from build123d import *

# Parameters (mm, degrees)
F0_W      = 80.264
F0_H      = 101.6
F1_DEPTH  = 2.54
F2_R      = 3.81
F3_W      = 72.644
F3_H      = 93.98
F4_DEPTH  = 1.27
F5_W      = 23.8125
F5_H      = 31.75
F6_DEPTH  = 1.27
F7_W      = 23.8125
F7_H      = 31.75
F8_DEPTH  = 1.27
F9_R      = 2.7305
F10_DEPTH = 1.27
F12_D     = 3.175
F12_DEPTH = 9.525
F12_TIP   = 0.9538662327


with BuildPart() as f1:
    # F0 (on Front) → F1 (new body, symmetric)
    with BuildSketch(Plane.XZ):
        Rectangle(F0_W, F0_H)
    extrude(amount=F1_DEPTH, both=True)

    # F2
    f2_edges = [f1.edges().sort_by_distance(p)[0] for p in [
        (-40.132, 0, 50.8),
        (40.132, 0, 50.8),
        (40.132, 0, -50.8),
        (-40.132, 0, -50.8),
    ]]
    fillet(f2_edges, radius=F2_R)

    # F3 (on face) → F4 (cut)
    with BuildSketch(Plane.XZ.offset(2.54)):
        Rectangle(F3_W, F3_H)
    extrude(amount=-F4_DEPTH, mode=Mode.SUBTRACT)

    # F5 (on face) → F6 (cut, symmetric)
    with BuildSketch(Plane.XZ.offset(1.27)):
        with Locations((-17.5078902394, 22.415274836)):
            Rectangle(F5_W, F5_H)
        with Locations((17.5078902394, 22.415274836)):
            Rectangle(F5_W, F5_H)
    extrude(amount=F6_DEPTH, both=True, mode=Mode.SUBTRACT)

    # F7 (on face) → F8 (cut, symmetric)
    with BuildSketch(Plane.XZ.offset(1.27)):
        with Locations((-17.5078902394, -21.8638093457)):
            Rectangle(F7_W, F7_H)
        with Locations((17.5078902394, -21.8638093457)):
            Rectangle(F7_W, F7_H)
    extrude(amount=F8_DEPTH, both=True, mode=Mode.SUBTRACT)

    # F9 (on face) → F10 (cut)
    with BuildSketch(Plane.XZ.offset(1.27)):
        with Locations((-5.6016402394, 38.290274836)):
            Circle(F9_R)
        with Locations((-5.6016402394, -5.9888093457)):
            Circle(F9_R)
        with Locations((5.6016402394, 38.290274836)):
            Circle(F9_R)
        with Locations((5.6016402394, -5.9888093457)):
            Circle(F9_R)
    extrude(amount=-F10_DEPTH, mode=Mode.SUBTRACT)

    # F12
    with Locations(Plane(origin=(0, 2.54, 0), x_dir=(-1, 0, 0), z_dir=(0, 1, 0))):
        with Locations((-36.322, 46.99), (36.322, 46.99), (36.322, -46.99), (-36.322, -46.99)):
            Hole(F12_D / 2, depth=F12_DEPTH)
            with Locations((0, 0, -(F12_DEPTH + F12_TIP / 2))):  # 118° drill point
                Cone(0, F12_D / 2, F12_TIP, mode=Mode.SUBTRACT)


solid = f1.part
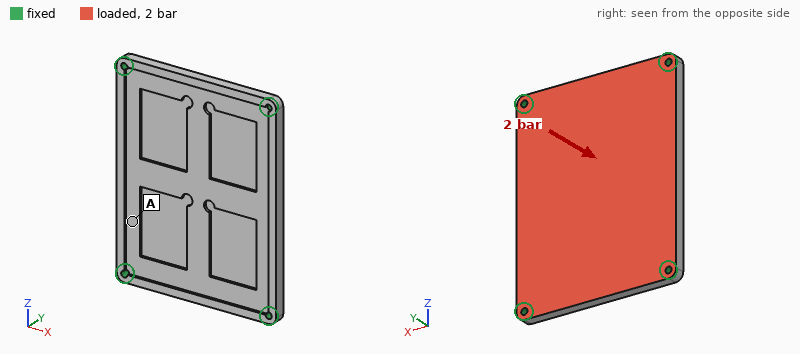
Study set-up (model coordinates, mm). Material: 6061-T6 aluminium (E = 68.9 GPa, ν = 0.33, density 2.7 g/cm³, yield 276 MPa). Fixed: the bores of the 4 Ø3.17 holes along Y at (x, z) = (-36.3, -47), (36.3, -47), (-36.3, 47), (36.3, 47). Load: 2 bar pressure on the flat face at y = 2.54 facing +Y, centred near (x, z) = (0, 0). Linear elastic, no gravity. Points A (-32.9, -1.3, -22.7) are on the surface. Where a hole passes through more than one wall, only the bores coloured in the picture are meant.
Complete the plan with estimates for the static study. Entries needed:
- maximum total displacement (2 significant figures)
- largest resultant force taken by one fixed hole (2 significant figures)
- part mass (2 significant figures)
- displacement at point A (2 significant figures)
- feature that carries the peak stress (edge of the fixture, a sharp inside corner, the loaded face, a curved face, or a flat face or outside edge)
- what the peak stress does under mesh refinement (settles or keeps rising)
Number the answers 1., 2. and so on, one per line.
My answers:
1. 0.28 mm
2. 580 N
3. 77 g
4. 0.13 mm
5. edge of the fixture
6. keeps rising
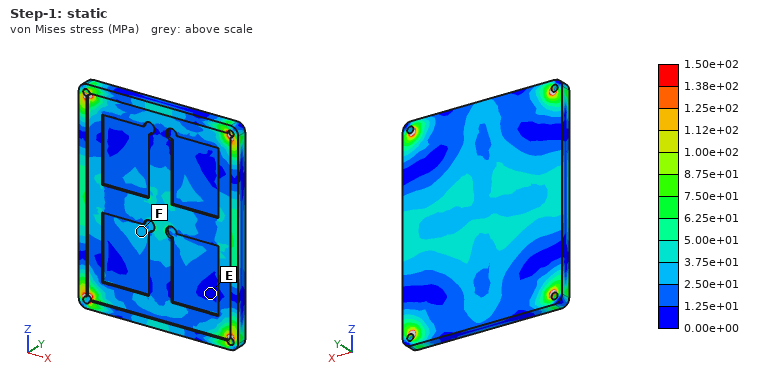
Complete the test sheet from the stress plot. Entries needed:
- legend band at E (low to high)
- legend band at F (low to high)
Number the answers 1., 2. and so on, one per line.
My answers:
1. 0.00e+00 to 1.25e+01 MPa
2. 2.50e+01 to 3.75e+01 MPa
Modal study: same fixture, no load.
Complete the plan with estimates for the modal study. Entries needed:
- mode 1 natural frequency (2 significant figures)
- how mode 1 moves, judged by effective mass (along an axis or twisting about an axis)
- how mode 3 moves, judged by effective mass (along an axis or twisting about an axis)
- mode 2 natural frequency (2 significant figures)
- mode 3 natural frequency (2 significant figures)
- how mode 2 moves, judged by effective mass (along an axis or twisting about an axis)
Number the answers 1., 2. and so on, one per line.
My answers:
1. 1700 Hz
2. along Y
3. twisting about X
4. 2700 Hz
5. 3600 Hz
6. twisting about Z
